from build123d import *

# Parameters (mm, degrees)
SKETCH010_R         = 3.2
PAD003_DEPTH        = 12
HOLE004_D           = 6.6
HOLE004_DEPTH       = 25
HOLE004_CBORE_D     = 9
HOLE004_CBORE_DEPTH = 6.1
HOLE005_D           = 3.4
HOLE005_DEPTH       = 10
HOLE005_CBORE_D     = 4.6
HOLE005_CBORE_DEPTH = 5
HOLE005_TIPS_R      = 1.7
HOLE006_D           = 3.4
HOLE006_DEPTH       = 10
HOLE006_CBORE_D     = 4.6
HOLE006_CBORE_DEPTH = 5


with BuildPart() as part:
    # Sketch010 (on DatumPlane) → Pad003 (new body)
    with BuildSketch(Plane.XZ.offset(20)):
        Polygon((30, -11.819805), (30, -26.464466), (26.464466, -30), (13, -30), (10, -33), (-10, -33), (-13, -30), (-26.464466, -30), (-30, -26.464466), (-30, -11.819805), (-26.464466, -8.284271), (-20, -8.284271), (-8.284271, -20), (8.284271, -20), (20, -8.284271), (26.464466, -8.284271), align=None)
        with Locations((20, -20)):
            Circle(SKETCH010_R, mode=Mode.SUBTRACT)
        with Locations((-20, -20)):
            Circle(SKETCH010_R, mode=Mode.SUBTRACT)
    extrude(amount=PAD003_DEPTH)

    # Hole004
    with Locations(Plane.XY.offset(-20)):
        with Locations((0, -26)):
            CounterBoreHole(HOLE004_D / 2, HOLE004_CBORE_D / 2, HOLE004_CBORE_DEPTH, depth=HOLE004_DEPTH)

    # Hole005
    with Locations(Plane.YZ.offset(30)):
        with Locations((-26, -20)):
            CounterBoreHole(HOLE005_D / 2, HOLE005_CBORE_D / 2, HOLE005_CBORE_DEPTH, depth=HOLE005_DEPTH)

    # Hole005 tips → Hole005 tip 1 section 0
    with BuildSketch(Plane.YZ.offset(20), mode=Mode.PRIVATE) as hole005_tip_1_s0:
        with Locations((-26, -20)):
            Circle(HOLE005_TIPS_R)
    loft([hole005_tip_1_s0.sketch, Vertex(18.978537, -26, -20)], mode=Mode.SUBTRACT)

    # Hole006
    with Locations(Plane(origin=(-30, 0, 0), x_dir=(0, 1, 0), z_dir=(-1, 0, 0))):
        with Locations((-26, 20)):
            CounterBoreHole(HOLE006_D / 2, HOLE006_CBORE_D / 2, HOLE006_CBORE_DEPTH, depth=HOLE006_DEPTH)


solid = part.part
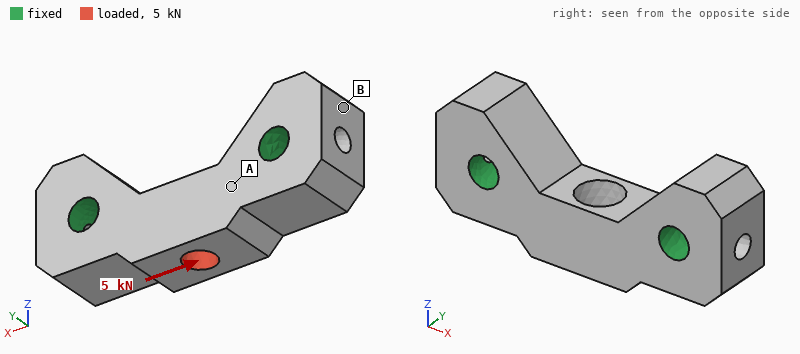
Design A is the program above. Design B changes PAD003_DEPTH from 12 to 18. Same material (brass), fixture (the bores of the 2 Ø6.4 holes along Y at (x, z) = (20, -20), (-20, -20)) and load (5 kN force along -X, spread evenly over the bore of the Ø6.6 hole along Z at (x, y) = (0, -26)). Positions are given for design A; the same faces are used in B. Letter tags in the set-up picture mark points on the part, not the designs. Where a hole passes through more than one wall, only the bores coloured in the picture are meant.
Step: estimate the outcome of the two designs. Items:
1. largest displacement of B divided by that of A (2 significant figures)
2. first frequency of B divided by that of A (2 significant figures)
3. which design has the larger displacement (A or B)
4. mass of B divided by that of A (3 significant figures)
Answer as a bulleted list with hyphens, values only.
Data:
- 0.87
- 1.1
- A
- 1.54
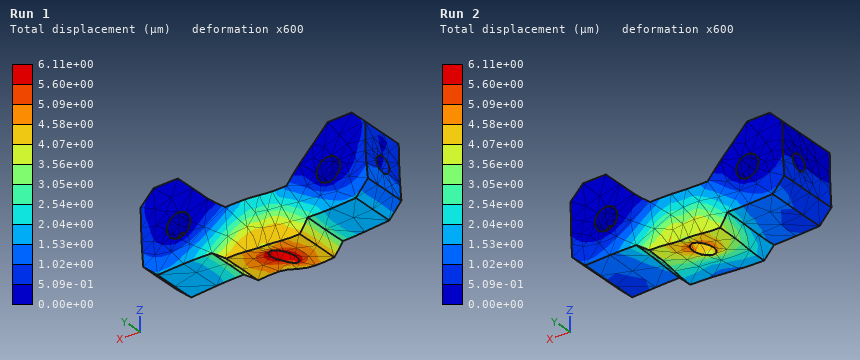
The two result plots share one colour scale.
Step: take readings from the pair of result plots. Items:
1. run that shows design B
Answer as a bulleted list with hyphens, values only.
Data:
- Run 2
